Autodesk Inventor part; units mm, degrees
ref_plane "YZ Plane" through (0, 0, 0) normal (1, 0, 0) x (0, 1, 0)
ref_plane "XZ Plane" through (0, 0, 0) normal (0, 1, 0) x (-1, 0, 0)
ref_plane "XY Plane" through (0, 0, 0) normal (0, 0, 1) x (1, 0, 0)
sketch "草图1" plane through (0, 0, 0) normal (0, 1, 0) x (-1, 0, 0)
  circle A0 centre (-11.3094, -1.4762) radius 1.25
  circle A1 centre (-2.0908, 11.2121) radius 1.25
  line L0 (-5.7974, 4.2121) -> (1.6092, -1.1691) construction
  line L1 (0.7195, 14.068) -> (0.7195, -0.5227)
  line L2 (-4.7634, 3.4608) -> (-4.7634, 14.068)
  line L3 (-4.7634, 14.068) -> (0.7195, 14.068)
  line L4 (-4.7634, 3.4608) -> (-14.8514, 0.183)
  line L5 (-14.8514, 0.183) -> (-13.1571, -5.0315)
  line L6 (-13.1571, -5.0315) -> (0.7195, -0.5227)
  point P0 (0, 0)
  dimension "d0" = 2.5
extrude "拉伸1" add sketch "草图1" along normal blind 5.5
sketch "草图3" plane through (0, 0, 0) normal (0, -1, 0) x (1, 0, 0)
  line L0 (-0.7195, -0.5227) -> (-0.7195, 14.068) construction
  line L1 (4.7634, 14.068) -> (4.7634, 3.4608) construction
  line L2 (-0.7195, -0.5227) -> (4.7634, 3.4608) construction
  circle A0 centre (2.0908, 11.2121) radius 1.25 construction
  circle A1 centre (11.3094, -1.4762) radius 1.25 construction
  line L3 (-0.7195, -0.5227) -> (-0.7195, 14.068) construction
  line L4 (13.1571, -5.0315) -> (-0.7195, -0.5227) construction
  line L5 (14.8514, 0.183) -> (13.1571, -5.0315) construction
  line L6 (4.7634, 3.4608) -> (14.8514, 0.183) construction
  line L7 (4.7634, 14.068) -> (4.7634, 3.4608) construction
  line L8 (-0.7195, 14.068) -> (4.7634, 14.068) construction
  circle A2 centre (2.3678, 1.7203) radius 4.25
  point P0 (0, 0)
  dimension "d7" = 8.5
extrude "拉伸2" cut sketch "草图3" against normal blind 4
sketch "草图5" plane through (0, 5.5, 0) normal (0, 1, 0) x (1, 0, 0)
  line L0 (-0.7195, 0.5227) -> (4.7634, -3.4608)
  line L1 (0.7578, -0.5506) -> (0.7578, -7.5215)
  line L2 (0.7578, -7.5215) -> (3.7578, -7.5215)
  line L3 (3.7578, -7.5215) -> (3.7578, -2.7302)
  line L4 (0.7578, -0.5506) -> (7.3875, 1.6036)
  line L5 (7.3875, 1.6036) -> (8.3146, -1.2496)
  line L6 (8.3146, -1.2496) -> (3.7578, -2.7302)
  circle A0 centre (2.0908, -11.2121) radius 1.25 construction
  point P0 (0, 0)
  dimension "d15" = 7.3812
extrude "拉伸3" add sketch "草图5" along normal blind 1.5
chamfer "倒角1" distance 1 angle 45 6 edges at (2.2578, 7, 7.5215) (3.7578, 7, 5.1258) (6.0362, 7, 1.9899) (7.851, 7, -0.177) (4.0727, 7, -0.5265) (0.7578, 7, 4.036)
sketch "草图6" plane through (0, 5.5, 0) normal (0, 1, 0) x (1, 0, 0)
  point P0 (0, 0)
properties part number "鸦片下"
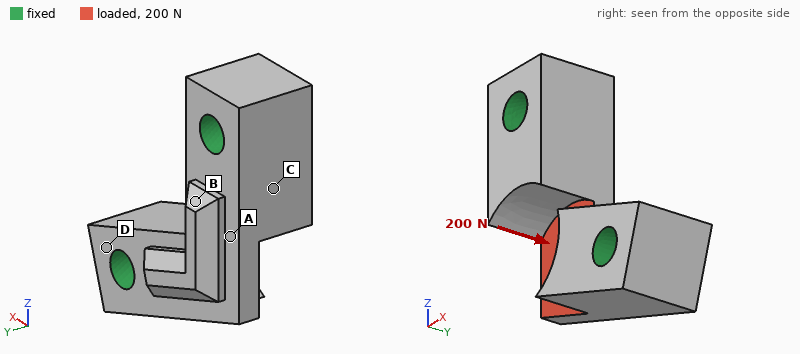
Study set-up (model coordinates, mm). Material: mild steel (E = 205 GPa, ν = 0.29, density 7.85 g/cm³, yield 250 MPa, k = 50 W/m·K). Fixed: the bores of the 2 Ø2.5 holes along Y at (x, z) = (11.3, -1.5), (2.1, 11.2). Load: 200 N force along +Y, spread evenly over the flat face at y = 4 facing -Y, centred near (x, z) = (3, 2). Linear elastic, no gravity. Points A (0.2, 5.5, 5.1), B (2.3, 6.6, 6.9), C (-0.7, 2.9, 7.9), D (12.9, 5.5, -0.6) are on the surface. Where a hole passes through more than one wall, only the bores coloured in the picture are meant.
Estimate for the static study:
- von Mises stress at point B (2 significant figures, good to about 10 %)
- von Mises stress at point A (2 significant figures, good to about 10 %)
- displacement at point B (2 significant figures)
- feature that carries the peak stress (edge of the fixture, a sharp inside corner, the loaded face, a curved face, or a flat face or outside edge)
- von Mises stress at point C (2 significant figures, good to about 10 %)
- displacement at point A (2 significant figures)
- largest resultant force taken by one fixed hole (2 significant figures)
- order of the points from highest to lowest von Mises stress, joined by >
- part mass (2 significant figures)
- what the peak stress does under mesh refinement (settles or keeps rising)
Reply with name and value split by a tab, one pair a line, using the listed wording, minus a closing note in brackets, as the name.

von Mises stress at point B	11 MPa
von Mises stress at point A	34 MPa
displacement at point B	1.0 µm
feature that carries the peak stress	a sharp inside corner
von Mises stress at point C	19 MPa
displacement at point A	1.4 µm
largest resultant force taken by one fixed hole	110 N
order of the points from highest to lowest von Mises stress, joined by >	A > C > B > D
part mass	4.4 g
what the peak stress does under mesh refinement	keeps rising
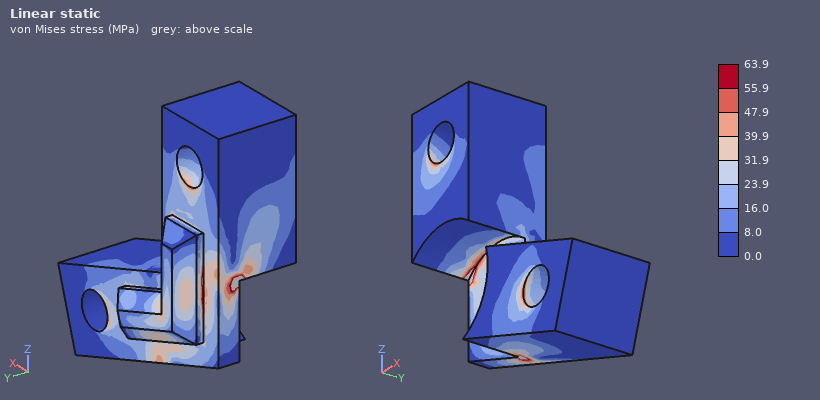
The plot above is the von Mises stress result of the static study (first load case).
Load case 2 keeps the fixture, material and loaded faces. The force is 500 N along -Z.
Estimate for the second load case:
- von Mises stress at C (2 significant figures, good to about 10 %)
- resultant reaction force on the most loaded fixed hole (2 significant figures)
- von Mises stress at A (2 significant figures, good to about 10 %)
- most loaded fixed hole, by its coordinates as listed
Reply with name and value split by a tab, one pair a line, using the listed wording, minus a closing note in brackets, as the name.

von Mises stress at C	9.6 MPa
resultant reaction force on the most loaded fixed hole	390 N
von Mises stress at A	15 MPa
most loaded fixed hole, by its coordinates as listed	(2.1, 11.2)
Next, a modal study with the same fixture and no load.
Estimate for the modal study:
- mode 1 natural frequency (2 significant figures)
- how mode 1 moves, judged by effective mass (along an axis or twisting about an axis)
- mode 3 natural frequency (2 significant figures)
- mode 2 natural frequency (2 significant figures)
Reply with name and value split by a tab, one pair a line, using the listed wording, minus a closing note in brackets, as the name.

mode 1 natural frequency	48 kHz
how mode 1 moves, judged by effective mass	along Y
mode 3 natural frequency	94 kHz
mode 2 natural frequency	89 kHz
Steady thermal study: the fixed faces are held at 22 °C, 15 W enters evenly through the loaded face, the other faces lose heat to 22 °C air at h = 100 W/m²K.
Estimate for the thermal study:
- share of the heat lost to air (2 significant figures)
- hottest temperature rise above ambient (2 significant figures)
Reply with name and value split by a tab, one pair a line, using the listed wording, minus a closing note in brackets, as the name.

share of the heat lost to air	5.8 %
hottest temperature rise above ambient	79 K
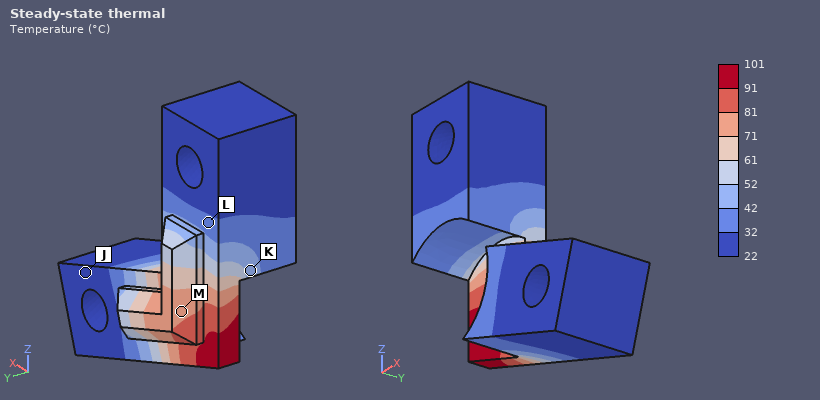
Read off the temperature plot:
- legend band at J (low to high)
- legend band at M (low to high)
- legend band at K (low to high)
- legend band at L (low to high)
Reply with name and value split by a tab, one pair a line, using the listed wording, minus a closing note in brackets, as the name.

legend band at J	22 to 32 °C
legend band at M	71 to 81 °C
legend band at K	42 to 52 °C
legend band at L	32 to 42 °C
